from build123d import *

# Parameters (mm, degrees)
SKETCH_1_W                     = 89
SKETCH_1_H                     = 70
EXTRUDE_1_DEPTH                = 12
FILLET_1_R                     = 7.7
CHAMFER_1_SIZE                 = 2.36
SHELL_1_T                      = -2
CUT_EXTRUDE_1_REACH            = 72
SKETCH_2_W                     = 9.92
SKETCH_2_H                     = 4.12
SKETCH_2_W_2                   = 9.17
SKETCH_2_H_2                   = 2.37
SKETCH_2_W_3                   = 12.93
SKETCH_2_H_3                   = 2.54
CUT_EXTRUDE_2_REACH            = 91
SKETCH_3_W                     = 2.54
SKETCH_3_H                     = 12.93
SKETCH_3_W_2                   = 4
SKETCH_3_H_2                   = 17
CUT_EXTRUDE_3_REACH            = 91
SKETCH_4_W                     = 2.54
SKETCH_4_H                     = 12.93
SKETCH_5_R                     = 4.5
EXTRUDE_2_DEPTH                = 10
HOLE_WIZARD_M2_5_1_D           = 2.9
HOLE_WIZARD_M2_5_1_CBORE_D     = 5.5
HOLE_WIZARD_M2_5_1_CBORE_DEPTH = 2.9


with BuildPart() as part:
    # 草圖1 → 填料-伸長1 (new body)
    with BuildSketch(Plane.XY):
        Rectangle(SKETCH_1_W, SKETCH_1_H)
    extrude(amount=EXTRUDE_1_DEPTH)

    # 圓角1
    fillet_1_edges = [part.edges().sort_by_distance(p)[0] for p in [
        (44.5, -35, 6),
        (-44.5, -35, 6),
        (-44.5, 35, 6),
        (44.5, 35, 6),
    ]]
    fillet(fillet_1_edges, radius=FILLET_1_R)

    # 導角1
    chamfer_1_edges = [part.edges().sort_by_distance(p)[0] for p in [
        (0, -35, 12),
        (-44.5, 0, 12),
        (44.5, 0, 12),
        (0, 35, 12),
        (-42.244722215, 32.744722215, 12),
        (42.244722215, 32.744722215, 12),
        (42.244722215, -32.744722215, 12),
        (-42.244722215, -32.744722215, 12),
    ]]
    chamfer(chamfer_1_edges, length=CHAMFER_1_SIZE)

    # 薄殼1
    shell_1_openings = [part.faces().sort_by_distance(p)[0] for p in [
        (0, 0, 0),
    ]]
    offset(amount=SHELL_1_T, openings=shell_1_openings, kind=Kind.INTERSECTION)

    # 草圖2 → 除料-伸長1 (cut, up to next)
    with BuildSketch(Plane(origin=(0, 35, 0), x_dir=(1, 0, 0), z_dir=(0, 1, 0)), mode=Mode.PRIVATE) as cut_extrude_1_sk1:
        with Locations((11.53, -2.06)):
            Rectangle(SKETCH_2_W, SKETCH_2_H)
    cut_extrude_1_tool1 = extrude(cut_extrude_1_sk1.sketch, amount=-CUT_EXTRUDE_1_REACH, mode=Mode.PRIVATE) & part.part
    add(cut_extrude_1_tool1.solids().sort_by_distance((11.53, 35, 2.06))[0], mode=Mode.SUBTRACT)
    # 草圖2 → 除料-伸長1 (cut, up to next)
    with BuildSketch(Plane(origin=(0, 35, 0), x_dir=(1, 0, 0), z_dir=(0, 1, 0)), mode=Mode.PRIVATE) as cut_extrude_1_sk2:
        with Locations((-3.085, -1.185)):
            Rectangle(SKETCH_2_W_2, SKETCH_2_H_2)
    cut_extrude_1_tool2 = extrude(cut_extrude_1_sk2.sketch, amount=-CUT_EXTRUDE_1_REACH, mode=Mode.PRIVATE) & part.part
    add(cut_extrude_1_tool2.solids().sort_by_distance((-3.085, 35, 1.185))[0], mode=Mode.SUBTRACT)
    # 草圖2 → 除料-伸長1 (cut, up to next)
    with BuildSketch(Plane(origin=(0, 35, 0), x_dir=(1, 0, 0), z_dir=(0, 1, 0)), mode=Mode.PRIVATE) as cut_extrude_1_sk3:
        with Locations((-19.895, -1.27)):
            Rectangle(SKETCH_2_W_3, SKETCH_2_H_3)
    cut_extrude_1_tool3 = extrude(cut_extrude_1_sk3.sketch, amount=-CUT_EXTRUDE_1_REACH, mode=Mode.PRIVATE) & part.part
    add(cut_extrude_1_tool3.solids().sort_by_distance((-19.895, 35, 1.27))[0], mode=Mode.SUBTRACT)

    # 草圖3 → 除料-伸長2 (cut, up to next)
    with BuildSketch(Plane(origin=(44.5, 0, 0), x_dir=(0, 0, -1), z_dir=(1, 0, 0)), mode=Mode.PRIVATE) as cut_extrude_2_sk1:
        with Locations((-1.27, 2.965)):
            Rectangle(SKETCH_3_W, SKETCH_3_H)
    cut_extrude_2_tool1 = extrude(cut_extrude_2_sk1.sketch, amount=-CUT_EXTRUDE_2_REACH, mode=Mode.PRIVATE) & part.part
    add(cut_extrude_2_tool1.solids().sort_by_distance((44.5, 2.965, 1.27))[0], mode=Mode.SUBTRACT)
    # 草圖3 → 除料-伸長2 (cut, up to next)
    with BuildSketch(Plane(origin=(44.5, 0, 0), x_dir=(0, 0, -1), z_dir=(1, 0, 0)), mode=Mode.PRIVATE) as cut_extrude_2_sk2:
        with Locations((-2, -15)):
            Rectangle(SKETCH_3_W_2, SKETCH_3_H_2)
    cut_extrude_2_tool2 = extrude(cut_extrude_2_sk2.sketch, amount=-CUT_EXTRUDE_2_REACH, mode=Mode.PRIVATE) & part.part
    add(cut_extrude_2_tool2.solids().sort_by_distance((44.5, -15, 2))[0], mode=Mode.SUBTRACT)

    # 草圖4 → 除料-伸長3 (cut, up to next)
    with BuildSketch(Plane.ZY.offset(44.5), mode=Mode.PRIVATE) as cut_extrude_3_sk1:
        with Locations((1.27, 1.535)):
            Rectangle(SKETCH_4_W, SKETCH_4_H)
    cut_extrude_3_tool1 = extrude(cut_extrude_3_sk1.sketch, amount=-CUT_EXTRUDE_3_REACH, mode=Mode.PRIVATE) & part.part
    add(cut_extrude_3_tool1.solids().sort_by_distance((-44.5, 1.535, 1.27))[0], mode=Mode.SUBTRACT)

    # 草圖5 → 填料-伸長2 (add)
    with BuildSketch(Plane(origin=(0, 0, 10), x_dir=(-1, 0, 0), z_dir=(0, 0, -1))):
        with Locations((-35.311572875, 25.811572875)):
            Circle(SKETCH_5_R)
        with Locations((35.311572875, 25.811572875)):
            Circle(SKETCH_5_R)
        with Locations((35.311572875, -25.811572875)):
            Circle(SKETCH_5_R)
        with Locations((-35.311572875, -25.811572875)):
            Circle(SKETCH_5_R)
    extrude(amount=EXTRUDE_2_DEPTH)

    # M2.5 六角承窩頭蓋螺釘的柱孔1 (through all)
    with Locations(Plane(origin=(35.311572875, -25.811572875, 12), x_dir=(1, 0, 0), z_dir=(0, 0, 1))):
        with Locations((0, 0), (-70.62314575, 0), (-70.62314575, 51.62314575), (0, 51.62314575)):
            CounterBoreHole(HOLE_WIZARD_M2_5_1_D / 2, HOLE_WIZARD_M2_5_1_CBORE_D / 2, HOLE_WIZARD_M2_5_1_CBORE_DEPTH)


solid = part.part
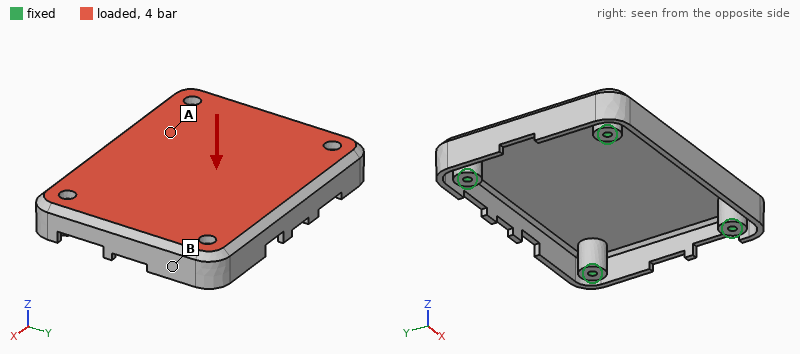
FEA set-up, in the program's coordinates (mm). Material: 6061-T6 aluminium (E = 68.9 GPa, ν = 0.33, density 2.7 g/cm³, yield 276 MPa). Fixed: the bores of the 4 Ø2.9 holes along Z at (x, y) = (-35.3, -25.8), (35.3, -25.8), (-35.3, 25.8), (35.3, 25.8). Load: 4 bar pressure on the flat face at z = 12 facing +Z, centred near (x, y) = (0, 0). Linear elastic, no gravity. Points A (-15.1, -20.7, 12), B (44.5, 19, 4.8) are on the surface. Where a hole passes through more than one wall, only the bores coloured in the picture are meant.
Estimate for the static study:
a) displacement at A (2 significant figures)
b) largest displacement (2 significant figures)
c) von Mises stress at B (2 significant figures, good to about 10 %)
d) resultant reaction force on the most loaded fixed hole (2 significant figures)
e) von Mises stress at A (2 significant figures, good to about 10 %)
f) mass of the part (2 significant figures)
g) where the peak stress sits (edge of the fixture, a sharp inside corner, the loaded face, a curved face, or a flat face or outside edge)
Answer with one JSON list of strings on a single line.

["0.21 mm", "0.49 mm", "23 MPa", "670 N", "56 MPa", "52 g", "the loaded face"]
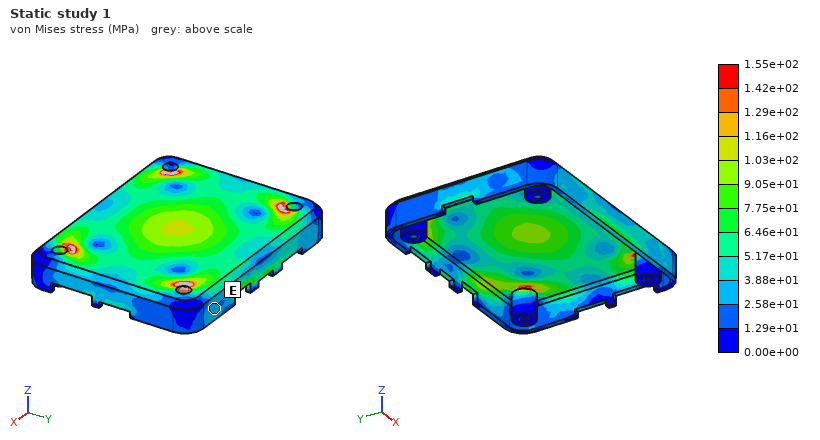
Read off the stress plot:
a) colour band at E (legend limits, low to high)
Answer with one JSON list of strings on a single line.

["2.58e+01 to 3.88e+01 MPa"]
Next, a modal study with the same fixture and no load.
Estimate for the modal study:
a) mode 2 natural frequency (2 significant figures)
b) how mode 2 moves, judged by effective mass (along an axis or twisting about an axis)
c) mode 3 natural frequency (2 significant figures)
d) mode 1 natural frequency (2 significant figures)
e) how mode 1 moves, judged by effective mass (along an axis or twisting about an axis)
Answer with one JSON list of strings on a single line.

["4500 Hz", "twisting about X", "5000 Hz", "2400 Hz", "along Z"]
